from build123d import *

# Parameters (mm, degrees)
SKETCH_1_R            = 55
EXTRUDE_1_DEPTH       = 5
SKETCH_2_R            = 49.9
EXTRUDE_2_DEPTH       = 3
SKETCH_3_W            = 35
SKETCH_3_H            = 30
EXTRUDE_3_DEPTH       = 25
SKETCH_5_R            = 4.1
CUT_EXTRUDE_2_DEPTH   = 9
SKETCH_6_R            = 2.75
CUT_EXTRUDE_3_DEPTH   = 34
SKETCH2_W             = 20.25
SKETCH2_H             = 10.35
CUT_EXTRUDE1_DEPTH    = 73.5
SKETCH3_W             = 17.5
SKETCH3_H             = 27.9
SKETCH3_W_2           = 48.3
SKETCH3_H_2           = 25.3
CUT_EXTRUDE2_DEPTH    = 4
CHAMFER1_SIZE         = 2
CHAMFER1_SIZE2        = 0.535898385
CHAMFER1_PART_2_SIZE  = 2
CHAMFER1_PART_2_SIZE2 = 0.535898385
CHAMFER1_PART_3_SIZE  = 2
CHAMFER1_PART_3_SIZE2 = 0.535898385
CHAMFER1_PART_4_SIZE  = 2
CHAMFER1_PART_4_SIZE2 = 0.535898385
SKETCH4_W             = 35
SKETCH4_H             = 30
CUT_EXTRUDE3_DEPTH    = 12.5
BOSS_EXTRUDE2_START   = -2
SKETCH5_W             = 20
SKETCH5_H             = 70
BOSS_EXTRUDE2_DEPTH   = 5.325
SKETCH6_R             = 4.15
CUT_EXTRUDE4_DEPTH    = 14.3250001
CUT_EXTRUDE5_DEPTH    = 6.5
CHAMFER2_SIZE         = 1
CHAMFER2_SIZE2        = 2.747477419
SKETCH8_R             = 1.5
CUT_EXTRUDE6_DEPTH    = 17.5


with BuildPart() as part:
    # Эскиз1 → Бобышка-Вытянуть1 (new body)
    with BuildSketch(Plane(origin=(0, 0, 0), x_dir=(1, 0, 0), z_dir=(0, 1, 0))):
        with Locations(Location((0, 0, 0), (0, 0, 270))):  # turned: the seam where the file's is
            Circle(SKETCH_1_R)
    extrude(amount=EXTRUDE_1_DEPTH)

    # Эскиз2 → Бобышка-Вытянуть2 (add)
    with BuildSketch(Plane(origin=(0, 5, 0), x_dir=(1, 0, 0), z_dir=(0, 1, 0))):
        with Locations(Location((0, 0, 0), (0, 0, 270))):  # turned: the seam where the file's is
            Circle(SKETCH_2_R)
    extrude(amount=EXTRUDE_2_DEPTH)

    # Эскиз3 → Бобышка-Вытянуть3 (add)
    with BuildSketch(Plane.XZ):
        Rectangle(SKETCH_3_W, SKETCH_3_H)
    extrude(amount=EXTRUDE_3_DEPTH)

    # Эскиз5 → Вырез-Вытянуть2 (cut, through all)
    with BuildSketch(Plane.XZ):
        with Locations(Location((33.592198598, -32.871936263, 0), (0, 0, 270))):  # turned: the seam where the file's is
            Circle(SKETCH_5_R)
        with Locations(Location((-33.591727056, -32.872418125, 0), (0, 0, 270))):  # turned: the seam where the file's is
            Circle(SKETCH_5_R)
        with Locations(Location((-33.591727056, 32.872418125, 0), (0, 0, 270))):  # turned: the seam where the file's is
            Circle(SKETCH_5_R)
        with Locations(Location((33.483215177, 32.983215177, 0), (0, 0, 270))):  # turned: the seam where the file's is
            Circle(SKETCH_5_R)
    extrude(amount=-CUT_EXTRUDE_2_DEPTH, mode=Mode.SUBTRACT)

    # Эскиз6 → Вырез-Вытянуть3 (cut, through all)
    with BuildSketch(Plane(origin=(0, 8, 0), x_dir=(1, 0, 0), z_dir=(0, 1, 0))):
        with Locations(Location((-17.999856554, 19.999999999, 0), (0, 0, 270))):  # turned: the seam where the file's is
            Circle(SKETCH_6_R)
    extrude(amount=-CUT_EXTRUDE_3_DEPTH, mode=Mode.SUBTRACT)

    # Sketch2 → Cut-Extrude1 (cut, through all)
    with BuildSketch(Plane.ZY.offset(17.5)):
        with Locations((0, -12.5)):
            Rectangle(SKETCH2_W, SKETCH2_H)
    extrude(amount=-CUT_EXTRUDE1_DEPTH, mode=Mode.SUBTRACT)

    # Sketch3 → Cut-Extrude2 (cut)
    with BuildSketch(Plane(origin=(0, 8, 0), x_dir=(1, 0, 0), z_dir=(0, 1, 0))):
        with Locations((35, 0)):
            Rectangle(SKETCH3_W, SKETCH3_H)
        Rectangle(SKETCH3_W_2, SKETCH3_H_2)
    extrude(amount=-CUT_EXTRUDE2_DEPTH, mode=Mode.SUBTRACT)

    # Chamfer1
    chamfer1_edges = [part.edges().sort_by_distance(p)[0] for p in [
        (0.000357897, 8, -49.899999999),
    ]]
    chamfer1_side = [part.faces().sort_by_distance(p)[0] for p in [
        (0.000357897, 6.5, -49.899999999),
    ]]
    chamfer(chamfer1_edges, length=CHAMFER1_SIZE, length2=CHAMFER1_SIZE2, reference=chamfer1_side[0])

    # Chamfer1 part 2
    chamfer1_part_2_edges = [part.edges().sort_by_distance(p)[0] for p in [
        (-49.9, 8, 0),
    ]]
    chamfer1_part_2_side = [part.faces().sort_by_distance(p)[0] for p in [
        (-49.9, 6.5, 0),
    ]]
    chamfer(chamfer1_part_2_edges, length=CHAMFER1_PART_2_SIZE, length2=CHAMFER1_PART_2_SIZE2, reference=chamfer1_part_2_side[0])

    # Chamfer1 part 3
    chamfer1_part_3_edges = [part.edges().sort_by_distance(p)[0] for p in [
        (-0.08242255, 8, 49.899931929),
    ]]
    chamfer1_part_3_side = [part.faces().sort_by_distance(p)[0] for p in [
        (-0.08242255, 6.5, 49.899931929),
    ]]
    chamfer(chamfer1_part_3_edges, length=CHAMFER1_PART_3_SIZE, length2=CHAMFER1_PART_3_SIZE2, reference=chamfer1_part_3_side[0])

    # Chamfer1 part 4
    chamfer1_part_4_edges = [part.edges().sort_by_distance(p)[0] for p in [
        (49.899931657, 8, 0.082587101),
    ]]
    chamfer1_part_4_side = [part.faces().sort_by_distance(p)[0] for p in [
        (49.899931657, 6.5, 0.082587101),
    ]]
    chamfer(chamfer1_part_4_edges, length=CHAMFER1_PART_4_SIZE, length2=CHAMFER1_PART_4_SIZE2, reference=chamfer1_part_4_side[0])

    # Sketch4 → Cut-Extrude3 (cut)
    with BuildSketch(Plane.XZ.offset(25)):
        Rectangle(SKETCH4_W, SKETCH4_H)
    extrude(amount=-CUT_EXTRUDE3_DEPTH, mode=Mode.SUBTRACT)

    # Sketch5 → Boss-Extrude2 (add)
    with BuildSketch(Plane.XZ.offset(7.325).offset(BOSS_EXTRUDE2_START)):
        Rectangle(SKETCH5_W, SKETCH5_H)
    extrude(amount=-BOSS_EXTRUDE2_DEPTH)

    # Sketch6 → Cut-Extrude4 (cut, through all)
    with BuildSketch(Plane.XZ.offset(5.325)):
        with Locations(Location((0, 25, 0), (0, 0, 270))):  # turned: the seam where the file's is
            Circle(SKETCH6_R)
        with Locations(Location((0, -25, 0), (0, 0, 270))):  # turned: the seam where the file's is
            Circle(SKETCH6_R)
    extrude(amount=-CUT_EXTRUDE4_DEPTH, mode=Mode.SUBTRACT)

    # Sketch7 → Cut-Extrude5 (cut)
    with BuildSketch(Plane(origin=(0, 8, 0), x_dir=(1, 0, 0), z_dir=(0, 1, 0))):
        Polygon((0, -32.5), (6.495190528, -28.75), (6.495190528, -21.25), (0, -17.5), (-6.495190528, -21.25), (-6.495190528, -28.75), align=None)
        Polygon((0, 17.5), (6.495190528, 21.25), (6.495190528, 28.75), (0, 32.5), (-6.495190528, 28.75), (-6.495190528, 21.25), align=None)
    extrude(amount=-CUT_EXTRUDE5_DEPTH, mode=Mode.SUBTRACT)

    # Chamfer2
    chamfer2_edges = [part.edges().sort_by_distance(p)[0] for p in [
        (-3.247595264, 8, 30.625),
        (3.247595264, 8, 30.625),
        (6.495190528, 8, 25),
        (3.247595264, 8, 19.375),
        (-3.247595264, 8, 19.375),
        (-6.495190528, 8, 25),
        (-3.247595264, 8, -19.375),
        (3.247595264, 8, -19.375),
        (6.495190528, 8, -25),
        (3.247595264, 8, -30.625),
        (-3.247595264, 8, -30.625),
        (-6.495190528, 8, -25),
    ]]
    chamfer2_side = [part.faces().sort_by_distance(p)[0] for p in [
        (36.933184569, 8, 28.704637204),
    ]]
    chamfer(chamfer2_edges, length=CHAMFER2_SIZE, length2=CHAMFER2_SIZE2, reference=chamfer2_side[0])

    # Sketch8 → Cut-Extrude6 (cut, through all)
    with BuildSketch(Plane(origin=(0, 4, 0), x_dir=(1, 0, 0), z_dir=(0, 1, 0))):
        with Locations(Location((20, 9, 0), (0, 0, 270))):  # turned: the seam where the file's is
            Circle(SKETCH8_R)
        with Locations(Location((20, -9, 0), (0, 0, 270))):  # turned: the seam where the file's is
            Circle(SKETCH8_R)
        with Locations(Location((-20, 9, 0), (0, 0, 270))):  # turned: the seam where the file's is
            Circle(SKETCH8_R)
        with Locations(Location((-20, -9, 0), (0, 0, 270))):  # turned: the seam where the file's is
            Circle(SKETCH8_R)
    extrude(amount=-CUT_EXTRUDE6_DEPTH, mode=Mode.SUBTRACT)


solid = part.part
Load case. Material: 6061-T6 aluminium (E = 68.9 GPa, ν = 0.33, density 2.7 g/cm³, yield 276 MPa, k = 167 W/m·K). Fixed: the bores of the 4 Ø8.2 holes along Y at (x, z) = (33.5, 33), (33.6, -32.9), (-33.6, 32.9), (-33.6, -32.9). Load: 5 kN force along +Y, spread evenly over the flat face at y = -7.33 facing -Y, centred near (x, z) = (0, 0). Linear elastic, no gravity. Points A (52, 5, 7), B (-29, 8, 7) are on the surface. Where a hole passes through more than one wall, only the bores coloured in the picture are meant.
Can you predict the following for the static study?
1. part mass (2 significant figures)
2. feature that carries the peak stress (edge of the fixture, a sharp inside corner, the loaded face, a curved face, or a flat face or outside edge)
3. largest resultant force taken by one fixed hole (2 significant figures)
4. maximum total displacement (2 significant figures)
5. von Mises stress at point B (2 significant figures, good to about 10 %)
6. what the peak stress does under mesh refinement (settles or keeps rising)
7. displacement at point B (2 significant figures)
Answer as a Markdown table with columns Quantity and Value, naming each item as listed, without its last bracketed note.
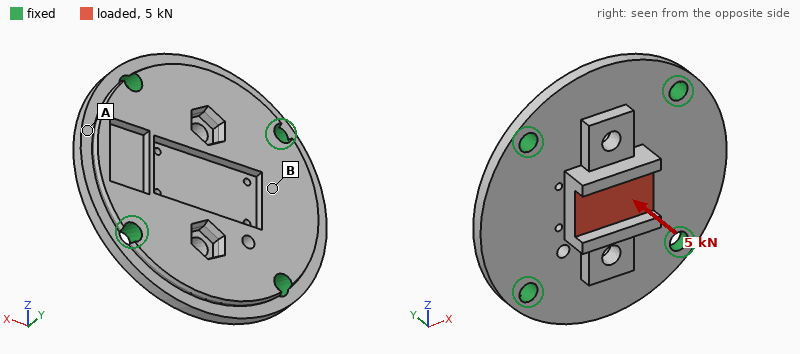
| Quantity | Value |
|---|---|
| part mass | 200 g |
| feature that carries the peak stress | edge of the fixture |
| largest resultant force taken by one fixed hole | 2.0 kN |
| maximum total displacement | 49 µm |
| von Mises stress at point B | 24 MPa |
| what the peak stress does under mesh refinement | keeps rising |
| displacement at point B | 26 µm |
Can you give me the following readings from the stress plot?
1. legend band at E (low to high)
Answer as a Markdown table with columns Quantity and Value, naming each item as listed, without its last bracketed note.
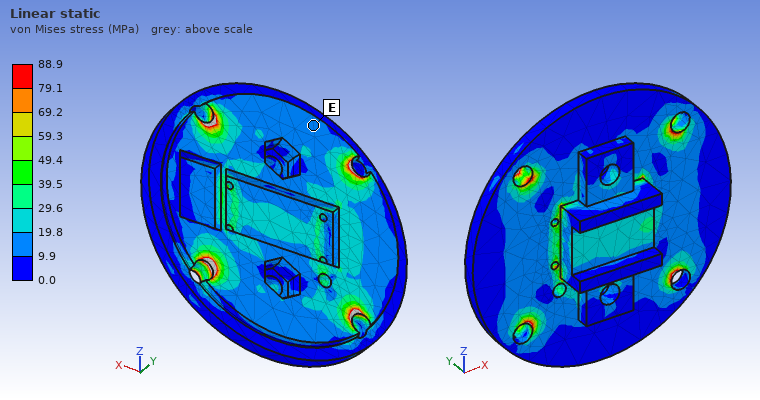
| Quantity | Value |
|---|---|
| legend band at E | 9.9 to 19.8 MPa |
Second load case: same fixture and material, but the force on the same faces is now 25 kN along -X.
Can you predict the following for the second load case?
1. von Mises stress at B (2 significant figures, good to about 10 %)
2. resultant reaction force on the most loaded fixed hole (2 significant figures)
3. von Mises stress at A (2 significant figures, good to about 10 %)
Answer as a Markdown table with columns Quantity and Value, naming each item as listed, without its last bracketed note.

| Quantity | Value |
|---|---|
| von Mises stress at B | 49 MPa |
| resultant reaction force on the most loaded fixed hole | 7.7 kN |
| von Mises stress at A | 31 MPa |
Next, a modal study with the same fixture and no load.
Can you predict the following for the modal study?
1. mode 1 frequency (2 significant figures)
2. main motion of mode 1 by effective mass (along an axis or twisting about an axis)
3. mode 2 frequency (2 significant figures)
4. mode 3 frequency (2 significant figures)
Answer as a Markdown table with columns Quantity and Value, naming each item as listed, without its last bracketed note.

| Quantity | Value |
|---|---|
| mode 1 frequency | 6500 Hz |
| main motion of mode 1 by effective mass | along Y |
| mode 2 frequency | 7800 Hz |
| mode 3 frequency | 8100 Hz |
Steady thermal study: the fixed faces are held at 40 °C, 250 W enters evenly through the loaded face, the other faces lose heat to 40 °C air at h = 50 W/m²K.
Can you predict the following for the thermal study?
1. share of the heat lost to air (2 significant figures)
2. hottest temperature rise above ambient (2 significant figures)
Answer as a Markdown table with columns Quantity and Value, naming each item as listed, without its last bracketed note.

| Quantity | Value |
|---|---|
| share of the heat lost to air | 10 % |
| hottest temperature rise above ambient | 66 K |
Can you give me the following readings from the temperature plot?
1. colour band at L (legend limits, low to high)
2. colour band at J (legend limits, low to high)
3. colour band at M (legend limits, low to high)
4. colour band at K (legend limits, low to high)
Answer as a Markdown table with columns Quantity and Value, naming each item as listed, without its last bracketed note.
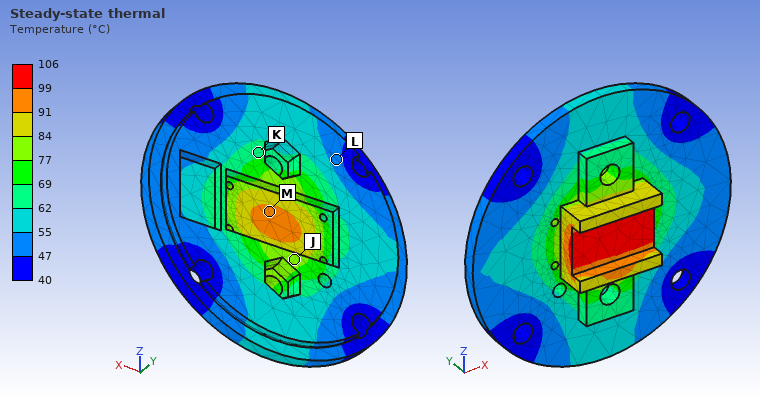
| Quantity | Value |
|---|---|
| colour band at L | 47 to 55 °C |
| colour band at J | 77 to 84 °C |
| colour band at M | 91 to 99 °C |
| colour band at K | 62 to 69 °C |
